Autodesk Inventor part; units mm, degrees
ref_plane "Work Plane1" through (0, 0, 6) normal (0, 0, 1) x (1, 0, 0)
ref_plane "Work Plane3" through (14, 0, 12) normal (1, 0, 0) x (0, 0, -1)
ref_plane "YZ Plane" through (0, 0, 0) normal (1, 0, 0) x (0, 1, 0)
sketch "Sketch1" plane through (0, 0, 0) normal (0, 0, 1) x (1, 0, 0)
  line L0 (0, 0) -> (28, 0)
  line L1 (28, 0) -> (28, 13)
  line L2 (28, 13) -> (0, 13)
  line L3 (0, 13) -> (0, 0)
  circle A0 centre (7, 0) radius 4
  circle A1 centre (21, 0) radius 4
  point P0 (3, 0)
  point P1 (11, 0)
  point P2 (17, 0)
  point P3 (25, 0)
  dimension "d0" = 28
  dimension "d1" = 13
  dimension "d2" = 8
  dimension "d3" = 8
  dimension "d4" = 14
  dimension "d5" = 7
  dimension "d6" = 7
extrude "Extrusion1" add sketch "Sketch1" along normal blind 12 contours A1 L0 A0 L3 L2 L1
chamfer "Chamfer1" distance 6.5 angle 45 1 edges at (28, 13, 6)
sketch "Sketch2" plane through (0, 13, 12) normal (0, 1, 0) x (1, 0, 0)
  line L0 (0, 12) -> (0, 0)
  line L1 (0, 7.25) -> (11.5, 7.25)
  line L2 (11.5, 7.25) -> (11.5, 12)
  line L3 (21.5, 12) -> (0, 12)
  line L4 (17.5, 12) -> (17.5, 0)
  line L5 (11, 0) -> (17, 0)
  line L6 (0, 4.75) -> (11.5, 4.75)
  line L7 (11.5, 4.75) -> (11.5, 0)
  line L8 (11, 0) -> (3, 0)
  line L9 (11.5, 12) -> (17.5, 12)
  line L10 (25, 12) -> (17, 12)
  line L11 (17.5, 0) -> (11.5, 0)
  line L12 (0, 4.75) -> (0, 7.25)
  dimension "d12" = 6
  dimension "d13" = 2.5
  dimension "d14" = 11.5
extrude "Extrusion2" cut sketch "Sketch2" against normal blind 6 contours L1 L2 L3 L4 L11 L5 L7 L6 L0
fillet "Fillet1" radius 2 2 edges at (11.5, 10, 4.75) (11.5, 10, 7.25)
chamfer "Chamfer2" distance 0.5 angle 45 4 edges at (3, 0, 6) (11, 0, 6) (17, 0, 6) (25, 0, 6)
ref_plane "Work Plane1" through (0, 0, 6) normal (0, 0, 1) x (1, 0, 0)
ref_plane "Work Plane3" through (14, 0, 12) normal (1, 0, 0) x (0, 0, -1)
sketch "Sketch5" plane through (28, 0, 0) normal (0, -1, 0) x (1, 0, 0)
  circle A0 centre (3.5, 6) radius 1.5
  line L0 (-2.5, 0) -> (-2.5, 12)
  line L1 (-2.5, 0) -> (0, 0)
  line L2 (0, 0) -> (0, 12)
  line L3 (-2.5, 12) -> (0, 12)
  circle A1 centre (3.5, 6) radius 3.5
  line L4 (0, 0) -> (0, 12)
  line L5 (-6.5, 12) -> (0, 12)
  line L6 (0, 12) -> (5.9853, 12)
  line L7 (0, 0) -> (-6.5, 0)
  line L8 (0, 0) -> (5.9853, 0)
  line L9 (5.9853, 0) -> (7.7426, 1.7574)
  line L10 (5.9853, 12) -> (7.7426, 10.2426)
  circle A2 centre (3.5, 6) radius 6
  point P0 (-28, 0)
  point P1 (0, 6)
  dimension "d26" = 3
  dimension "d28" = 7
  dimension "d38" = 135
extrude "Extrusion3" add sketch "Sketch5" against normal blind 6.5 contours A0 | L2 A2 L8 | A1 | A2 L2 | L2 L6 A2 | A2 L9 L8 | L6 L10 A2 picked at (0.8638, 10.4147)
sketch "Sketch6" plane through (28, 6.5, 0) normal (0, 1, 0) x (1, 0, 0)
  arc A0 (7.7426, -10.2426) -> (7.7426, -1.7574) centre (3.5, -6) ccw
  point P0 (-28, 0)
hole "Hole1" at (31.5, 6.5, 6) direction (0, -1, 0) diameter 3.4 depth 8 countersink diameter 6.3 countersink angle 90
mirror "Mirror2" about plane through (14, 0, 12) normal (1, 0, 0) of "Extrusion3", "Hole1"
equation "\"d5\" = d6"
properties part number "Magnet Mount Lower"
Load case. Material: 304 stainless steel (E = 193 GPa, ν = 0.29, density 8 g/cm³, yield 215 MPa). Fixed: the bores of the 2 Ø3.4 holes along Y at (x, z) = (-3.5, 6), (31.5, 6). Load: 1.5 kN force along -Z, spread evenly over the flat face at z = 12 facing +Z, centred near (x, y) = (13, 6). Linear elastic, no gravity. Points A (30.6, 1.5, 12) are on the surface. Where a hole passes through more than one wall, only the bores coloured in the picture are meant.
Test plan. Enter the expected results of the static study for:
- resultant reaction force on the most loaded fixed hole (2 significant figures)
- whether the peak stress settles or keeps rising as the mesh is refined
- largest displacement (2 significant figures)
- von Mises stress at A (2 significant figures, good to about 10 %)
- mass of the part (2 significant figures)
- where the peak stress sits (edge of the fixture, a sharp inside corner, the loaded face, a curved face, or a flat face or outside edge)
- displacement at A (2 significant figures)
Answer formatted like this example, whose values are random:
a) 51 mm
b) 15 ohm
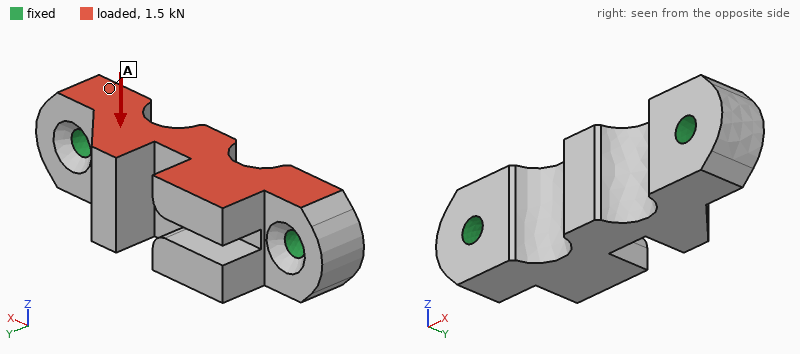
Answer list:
a) 790 N
b) keeps rising
c) 9.1 µm
d) 17 MPa
e) 32 g
f) edge of the fixture
g) 1.4 µm
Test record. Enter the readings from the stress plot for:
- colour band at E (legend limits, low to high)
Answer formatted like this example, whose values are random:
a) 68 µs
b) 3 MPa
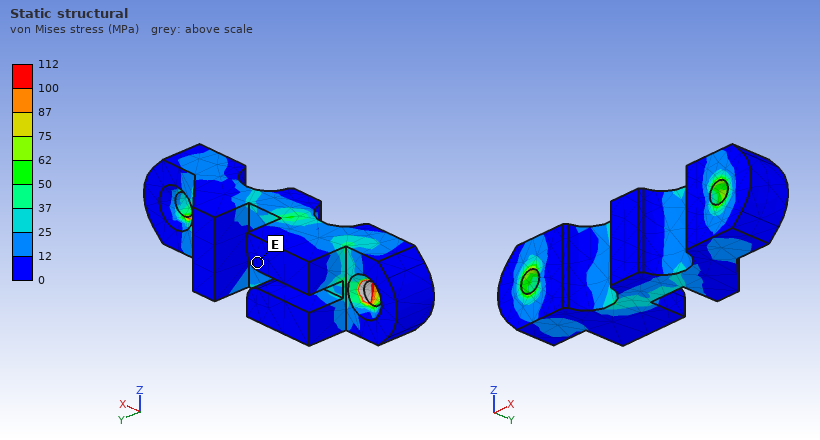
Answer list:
a) 0 to 12 MPa
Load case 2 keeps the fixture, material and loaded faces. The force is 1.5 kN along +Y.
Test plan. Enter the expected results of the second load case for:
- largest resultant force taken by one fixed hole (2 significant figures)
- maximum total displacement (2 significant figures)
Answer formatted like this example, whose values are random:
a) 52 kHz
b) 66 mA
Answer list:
a) 880 N
b) 15 µm
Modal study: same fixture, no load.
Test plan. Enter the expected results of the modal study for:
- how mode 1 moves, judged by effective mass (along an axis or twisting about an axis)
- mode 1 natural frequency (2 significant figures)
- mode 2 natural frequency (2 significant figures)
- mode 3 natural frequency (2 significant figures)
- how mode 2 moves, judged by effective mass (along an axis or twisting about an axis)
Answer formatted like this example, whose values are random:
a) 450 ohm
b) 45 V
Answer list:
a) along Y
b) 16 kHz
c) 17 kHz
d) 23 kHz
e) along Z
